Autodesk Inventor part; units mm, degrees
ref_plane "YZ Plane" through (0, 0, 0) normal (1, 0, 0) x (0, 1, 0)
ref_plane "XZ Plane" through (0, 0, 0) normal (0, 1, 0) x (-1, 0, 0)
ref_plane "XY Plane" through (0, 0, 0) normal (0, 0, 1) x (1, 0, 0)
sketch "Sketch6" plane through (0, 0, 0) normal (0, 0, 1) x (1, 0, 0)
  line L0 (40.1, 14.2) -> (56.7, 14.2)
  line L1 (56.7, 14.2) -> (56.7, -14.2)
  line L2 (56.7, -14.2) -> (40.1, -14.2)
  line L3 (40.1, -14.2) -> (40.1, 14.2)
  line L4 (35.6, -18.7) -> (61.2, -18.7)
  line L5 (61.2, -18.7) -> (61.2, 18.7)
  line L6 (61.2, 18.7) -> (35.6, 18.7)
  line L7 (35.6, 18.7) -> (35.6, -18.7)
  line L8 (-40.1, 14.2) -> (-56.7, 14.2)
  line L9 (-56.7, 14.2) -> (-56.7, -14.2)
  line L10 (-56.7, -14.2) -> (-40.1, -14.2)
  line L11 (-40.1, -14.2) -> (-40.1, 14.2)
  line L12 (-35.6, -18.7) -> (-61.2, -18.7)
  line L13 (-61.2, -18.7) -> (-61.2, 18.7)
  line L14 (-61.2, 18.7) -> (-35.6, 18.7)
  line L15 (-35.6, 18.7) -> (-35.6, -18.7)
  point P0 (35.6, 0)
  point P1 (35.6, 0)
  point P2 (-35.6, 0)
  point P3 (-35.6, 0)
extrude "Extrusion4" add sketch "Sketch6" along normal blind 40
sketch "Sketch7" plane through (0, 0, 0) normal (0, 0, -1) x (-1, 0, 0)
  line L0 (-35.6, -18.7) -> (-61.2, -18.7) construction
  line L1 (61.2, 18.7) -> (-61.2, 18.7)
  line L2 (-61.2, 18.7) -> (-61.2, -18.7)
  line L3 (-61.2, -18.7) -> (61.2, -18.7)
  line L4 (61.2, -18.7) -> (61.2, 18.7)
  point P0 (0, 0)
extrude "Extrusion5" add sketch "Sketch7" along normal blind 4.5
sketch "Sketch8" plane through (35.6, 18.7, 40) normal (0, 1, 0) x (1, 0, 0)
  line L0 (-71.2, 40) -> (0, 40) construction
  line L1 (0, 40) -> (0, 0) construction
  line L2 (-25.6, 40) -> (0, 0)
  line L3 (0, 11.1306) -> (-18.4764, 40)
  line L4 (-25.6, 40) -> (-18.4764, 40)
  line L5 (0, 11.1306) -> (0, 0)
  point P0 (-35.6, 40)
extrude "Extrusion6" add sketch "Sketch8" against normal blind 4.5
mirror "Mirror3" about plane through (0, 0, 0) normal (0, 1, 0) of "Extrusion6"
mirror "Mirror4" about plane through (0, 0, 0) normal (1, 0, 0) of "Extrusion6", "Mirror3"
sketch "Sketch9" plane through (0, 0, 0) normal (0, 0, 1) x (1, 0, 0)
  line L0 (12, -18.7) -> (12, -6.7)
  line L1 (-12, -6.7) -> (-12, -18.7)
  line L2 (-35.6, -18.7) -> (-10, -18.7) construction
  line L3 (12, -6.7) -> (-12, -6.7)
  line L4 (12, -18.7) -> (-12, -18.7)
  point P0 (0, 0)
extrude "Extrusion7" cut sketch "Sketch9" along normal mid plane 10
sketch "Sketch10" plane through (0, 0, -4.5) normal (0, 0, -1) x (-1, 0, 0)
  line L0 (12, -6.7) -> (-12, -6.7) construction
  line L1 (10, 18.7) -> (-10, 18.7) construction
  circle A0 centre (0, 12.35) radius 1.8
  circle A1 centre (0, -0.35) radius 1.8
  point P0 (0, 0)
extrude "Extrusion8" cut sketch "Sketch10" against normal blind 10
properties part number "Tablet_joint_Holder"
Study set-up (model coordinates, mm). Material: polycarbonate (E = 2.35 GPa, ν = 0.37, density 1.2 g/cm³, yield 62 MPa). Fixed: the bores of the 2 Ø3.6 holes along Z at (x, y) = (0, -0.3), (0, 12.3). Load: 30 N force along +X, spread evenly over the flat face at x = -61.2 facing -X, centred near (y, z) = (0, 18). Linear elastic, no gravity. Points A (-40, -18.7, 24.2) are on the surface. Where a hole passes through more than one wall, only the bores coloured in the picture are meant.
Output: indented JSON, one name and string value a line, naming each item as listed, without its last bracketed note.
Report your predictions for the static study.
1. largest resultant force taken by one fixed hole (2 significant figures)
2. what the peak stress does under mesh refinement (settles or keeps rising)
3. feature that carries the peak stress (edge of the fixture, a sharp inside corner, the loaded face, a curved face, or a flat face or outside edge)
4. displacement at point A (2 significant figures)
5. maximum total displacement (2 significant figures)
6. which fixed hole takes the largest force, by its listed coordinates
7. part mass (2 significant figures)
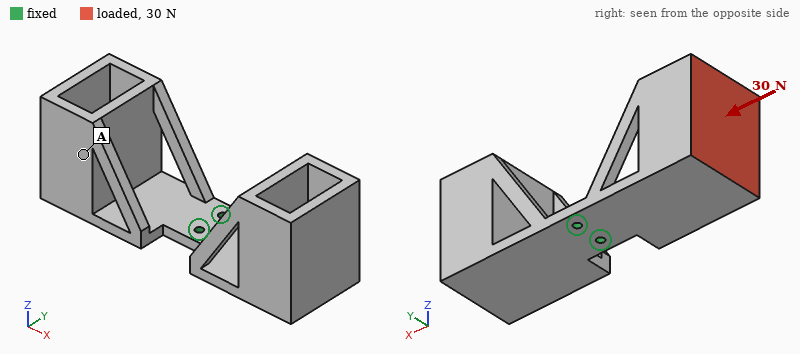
{
  "largest resultant force taken by one fixed hole": "27 N",
  "what the peak stress does under mesh refinement": "keeps rising",
  "feature that carries the peak stress": "edge of the fixture",
  "displacement at point A": "0.90 mm",
  "maximum total displacement": "1.6 mm",
  "which fixed hole takes the largest force, by its listed coordinates": "(0, -0.3)",
  "part mass": "75 g"
}
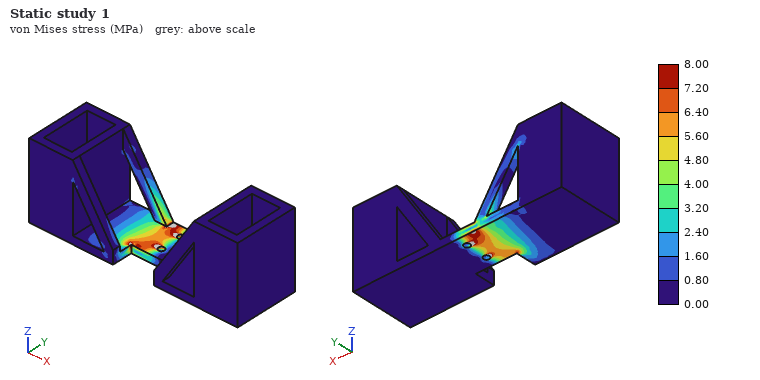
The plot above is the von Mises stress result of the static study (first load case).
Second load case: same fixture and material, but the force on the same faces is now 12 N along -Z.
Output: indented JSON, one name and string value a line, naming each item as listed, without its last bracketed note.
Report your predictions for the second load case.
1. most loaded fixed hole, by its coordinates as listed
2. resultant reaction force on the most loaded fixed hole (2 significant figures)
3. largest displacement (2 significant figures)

{
  "most loaded fixed hole, by its coordinates as listed": "(0, -0.3)",
  "resultant reaction force on the most loaded fixed hole": "10 N",
  "largest displacement": "1.6 mm"
}
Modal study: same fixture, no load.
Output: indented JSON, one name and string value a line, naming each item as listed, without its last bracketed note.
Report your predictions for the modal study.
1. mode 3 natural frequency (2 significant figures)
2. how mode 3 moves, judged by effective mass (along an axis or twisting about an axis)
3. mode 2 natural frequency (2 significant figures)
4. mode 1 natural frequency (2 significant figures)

{
  "mode 3 natural frequency": "230 Hz",
  "how mode 3 moves, judged by effective mass": "twisting about Z",
  "mode 2 natural frequency": "100 Hz",
  "mode 1 natural frequency": "100 Hz"
}
